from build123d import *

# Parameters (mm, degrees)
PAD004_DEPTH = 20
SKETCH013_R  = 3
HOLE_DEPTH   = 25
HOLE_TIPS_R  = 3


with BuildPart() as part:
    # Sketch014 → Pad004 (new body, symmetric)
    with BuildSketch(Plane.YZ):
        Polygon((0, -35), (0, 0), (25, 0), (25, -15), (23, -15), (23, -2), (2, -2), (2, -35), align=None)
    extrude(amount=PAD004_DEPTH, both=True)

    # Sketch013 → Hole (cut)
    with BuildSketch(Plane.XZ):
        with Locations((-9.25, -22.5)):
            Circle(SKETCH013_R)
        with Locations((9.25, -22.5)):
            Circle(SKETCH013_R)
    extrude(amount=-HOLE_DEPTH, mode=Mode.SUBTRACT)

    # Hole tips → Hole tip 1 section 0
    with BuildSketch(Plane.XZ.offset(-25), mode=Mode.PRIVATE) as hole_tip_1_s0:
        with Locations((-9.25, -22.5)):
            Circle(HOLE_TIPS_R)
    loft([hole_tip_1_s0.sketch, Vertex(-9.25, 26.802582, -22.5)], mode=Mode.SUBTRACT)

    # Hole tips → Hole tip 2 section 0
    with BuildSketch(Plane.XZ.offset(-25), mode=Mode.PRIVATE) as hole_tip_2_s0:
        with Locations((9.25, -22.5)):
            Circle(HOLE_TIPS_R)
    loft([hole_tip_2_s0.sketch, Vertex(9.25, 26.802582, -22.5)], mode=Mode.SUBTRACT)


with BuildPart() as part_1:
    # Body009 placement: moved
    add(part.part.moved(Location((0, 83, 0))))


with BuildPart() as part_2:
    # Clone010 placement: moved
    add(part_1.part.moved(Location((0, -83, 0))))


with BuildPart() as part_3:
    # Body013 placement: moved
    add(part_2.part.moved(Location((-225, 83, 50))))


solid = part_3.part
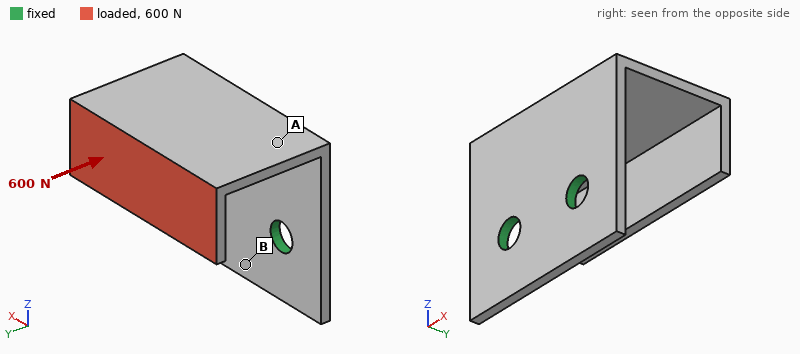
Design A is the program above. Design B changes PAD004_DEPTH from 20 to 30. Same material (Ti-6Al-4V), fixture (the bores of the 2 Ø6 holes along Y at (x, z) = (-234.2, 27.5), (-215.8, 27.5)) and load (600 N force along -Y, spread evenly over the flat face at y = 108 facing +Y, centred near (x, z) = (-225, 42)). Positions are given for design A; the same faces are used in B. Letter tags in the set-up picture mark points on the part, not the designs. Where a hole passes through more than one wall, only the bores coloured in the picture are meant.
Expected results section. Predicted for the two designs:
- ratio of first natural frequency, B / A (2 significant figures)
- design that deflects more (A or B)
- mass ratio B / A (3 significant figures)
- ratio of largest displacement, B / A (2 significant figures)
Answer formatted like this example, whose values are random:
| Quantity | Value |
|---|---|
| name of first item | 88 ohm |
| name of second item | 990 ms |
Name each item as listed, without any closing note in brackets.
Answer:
| Quantity | Value |
|---|---|
| ratio of first natural frequency, B / A | 0.96 |
| design that deflects more | A |
| mass ratio B / A | 1.51 |
| ratio of largest displacement, B / A | 0.71 |
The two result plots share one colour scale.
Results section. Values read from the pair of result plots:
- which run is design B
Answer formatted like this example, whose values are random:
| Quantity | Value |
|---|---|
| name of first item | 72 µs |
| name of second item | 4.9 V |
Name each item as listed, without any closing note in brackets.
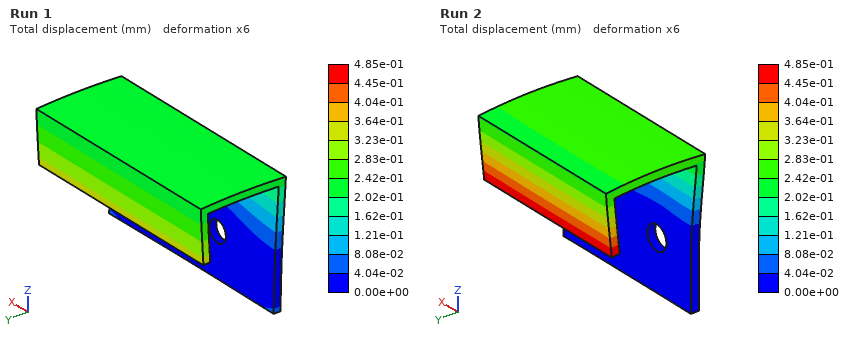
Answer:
| Quantity | Value |
|---|---|
| which run is design B | Run 1 |
